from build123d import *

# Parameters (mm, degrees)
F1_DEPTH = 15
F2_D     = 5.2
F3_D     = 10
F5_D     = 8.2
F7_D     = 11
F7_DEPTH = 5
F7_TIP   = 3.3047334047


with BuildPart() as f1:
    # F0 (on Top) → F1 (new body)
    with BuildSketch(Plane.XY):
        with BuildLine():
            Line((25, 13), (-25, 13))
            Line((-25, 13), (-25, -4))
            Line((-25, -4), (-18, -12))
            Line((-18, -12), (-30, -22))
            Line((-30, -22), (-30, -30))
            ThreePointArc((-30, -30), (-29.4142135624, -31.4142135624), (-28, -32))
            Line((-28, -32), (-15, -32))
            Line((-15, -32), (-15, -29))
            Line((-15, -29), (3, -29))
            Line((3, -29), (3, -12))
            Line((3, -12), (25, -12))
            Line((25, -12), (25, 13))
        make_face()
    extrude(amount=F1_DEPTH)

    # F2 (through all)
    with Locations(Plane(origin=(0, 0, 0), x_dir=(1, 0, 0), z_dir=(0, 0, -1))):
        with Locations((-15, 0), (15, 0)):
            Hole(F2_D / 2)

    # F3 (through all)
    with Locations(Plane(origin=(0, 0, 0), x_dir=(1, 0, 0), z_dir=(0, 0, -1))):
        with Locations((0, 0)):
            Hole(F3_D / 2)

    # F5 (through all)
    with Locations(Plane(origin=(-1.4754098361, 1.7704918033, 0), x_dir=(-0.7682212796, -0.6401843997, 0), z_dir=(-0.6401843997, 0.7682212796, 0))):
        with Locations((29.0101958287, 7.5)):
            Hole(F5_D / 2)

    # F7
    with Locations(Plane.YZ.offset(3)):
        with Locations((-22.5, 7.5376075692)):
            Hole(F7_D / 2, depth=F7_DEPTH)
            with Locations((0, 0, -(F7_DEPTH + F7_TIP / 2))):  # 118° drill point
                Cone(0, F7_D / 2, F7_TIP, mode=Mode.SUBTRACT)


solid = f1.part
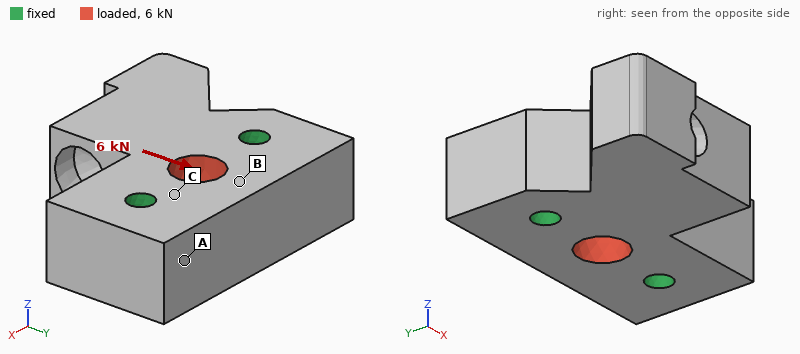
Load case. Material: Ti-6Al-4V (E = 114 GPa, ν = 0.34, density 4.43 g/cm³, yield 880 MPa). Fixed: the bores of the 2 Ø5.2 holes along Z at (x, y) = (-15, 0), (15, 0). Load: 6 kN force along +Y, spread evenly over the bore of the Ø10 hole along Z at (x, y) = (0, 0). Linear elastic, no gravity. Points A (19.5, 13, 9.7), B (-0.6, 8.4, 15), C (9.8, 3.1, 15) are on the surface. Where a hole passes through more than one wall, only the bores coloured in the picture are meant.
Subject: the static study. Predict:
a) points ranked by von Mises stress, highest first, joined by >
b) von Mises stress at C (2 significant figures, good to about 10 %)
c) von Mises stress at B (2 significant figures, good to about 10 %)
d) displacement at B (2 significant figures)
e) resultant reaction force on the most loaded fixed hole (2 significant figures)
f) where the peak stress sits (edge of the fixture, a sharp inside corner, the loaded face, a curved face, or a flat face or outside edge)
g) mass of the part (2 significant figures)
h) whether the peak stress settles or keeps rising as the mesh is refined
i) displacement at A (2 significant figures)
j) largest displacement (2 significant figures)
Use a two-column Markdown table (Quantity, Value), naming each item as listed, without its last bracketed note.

| Quantity | Value |
|---|---|
| points ranked by von Mises stress, highest first, joined by > | C > B > A |
| von Mises stress at C | 20 MPa |
| von Mises stress at B | 15 MPa |
| displacement at B | 3.3 µm |
| resultant reaction force on the most loaded fixed hole | 3.0 kN |
| where the peak stress sits | edge of the fixture |
| mass of the part | 100 g |
| whether the peak stress settles or keeps rising as the mesh is refined | keeps rising |
| displacement at A | 1.3 µm |
| largest displacement | 4.6 µm |
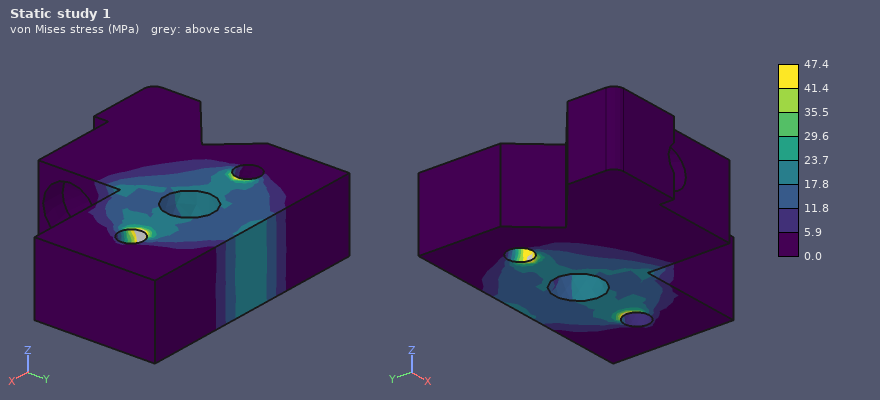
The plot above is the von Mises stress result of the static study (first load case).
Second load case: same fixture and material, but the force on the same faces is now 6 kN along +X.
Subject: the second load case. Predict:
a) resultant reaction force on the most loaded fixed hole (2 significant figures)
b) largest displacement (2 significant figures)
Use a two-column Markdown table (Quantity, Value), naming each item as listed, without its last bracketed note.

| Quantity | Value |
|---|---|
| resultant reaction force on the most loaded fixed hole | 3.0 kN |
| largest displacement | 1.7 µm |
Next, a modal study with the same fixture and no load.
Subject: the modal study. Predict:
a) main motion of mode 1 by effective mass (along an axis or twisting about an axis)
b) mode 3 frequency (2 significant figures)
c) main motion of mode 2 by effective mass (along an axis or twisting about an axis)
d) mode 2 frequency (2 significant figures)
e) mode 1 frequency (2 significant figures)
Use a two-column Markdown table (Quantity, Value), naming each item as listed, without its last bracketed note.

| Quantity | Value |
|---|---|
| main motion of mode 1 by effective mass | along Z |
| mode 3 frequency | 17 kHz |
| main motion of mode 2 by effective mass | along X |
| mode 2 frequency | 14 kHz |
| mode 1 frequency | 9300 Hz |
